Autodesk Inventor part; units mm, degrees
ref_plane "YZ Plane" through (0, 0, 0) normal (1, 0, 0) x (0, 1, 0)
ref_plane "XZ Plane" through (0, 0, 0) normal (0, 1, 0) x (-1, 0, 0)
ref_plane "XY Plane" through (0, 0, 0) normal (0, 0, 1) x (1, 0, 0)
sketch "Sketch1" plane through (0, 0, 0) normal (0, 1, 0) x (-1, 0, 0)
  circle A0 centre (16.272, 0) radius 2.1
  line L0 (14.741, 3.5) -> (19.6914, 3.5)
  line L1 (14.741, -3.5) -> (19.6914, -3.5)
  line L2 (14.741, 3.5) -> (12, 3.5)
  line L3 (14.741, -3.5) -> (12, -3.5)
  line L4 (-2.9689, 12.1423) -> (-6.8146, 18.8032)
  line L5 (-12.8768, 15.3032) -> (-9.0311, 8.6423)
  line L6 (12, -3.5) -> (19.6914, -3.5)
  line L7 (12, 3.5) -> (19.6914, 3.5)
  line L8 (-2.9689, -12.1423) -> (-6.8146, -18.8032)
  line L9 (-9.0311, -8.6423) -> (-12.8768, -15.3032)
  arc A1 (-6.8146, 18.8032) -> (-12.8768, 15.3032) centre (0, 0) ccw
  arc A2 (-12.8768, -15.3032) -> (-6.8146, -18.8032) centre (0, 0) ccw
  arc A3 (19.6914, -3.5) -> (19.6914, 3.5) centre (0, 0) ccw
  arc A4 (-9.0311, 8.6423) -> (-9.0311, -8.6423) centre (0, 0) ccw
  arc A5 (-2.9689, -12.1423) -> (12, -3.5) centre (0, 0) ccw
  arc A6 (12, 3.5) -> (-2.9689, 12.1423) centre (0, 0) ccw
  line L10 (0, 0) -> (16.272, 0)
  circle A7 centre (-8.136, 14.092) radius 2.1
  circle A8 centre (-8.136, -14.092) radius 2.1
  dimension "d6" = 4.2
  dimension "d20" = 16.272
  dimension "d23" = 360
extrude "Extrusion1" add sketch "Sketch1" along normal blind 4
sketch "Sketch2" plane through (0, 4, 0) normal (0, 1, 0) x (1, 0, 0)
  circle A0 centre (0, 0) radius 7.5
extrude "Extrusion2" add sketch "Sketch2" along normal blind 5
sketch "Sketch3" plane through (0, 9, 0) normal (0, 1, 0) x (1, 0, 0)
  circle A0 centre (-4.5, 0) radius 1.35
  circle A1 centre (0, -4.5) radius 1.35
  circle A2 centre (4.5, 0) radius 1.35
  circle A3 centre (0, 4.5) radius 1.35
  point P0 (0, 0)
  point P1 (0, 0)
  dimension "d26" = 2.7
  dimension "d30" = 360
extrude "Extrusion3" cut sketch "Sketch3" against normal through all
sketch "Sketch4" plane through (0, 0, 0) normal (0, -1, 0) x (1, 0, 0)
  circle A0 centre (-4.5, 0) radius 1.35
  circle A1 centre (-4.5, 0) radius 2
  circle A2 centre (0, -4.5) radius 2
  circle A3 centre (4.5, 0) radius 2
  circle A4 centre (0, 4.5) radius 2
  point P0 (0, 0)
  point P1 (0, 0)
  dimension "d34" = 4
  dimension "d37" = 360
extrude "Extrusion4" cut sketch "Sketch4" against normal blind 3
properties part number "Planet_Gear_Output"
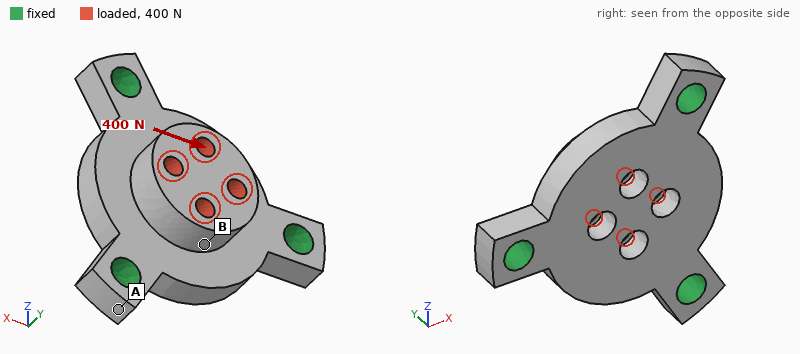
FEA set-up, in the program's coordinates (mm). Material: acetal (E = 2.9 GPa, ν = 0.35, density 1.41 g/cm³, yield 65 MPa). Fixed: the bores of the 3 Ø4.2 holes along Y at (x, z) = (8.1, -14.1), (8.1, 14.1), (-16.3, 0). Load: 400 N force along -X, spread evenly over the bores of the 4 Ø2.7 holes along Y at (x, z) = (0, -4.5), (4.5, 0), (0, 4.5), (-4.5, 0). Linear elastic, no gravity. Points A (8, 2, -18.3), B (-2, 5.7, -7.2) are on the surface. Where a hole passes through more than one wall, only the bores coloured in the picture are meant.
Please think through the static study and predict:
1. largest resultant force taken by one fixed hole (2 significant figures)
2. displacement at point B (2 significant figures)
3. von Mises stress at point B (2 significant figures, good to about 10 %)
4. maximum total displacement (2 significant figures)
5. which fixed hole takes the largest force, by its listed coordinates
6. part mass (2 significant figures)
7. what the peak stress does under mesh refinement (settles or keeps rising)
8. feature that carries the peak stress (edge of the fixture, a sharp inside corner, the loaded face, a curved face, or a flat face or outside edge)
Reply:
210 N
43 µm
3.8 MPa
80 µm
(-16.3, 0)
4.3 g
keeps rising
edge of the fixture
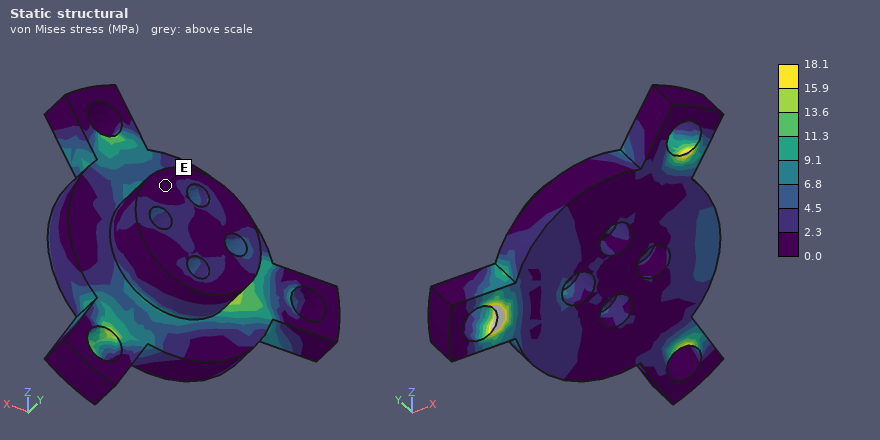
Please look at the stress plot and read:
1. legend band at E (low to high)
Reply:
0.0 to 2.3 MPa
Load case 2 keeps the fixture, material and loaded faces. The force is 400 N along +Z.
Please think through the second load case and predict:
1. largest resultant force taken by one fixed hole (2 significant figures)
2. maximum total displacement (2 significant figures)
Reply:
190 N
77 µm
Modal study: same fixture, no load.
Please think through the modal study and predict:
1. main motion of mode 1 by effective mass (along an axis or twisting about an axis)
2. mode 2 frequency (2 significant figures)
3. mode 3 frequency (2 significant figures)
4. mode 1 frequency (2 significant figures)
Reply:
along Y
7600 Hz
7600 Hz
5900 Hz
